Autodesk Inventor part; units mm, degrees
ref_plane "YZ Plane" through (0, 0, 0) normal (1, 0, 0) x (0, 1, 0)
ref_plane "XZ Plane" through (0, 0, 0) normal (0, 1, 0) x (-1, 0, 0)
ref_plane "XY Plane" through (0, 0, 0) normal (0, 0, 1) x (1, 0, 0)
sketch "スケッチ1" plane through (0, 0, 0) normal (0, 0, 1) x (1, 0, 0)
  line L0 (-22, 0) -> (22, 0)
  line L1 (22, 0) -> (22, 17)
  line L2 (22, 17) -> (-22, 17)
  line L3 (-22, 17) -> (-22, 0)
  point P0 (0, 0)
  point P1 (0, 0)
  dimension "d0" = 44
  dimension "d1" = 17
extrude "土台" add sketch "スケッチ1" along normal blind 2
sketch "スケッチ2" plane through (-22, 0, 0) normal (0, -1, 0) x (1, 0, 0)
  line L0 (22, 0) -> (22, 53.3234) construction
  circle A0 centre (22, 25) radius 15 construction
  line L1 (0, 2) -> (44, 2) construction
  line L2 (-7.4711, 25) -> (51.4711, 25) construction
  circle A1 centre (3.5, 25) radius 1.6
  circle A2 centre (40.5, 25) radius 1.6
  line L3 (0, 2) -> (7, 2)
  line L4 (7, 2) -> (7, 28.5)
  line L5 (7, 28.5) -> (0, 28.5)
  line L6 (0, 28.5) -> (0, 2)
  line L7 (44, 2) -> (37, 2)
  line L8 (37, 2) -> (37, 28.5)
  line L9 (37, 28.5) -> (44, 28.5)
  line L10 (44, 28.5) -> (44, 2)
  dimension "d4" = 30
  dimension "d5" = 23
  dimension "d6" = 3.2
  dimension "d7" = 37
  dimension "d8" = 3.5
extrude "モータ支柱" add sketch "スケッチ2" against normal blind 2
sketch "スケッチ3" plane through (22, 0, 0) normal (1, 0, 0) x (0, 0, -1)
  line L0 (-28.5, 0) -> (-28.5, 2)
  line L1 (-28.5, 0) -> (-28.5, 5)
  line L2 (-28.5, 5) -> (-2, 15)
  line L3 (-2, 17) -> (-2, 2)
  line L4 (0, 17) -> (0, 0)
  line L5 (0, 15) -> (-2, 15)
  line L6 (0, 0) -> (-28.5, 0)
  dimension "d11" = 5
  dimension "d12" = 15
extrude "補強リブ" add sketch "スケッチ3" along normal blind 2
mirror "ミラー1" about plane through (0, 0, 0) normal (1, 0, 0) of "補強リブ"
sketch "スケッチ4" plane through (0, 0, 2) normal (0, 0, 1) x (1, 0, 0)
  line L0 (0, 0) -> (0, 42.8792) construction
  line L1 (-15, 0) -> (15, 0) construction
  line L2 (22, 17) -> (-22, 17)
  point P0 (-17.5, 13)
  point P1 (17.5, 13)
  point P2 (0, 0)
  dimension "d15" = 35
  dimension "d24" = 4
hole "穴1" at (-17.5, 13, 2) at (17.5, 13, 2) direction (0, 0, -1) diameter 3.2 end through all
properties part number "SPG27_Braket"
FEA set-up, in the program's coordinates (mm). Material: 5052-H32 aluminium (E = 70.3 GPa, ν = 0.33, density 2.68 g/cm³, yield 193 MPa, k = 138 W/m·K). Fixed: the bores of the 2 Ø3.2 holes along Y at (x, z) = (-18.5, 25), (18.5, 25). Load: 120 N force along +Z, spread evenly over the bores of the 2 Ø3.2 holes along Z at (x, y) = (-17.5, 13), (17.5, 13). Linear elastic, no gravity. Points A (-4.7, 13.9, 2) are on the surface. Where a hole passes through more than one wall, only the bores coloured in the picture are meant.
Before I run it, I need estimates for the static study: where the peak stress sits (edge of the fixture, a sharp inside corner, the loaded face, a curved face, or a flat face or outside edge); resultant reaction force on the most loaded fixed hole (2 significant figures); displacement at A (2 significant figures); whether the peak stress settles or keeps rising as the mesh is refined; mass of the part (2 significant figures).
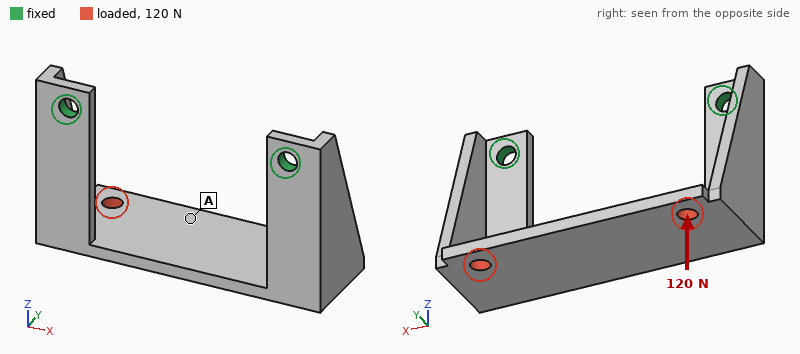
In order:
edge of the fixture
62 N
0.097 mm
keeps rising
9.0 g
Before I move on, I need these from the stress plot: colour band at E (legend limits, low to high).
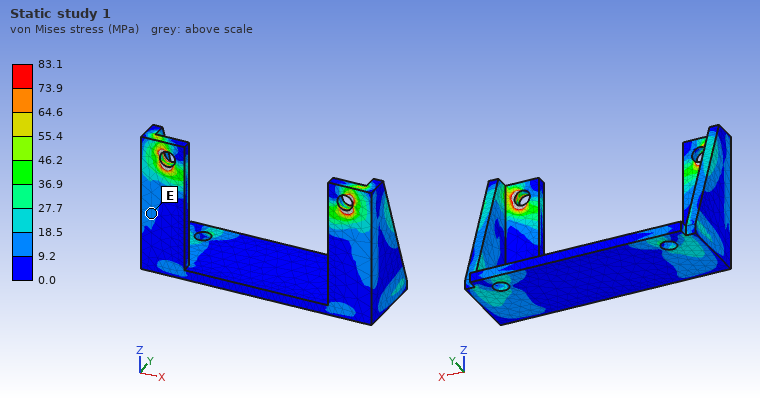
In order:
9.2 to 18.5 MPa
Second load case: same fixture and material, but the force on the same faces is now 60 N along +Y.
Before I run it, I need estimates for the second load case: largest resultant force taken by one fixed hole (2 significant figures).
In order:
31 N
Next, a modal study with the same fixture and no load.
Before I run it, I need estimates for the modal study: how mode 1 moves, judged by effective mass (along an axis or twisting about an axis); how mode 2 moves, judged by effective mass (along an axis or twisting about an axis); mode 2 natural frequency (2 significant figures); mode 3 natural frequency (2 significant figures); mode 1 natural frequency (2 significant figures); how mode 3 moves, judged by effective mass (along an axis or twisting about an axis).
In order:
along Y
along X
2400 Hz
4300 Hz
1800 Hz
along X
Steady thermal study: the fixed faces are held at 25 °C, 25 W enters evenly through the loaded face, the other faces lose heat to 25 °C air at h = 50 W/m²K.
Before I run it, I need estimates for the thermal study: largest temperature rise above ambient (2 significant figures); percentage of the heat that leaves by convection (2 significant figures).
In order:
75 K
31 %
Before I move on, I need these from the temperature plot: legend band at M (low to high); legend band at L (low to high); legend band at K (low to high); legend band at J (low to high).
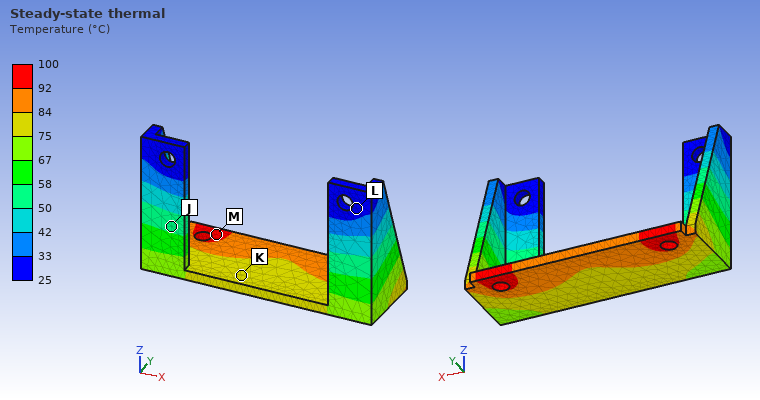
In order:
92 to 100 °C
25 to 33 °C
75 to 84 °C
50 to 58 °C
